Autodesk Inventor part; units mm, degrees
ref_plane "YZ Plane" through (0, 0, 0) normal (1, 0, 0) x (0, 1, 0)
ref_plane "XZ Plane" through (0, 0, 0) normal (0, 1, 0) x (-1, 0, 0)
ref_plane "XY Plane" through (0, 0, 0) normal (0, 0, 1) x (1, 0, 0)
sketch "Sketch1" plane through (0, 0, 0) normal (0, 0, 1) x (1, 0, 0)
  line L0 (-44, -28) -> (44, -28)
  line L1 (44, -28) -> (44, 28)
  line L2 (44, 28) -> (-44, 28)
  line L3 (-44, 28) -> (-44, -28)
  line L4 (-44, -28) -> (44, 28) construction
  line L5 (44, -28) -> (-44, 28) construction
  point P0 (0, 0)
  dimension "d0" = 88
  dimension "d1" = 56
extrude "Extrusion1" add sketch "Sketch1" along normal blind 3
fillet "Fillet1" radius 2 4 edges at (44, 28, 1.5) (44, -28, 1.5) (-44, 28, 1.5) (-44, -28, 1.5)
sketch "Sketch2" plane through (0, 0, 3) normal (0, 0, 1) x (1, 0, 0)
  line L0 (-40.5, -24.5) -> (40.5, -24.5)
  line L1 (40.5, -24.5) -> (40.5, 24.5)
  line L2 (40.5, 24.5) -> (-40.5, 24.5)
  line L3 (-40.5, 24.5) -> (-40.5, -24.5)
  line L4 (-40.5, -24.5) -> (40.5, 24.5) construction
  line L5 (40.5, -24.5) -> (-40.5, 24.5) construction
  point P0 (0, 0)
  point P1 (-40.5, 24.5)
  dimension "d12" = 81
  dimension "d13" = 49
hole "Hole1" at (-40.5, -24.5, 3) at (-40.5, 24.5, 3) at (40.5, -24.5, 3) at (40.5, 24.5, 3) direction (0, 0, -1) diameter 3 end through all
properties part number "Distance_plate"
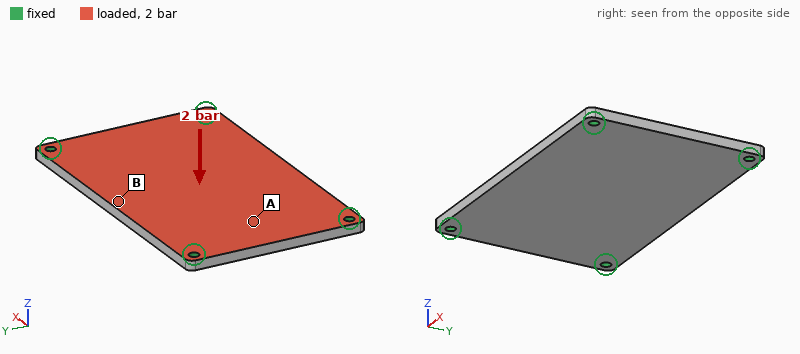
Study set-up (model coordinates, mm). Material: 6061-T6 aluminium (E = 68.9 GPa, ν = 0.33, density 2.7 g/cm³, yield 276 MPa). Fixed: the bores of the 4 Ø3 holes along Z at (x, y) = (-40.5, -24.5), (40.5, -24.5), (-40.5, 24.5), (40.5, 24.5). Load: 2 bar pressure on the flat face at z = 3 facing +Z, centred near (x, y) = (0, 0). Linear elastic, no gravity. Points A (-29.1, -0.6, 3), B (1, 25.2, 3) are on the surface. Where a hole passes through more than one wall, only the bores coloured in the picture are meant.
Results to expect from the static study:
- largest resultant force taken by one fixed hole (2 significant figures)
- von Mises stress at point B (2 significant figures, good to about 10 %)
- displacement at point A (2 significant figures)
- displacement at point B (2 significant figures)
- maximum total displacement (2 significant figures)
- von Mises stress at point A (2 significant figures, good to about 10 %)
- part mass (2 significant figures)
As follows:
240 N
50 MPa
0.10 mm
0.22 mm
0.23 mm
20 MPa
40 g
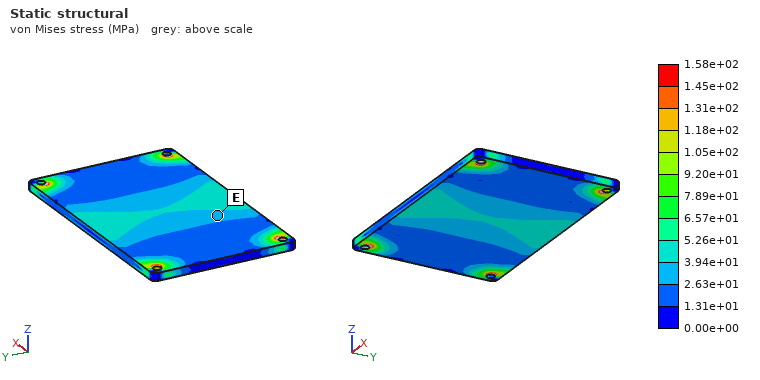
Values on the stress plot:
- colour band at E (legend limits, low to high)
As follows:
2.63e+01 to 3.94e+01 MPa
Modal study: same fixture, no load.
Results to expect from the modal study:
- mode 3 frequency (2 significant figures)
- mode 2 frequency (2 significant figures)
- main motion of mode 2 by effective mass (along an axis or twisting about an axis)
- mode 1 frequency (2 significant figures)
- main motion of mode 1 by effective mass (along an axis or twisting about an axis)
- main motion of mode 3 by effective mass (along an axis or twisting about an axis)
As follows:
4900 Hz
3200 Hz
twisting about X
1900 Hz
along Z
twisting about Y
